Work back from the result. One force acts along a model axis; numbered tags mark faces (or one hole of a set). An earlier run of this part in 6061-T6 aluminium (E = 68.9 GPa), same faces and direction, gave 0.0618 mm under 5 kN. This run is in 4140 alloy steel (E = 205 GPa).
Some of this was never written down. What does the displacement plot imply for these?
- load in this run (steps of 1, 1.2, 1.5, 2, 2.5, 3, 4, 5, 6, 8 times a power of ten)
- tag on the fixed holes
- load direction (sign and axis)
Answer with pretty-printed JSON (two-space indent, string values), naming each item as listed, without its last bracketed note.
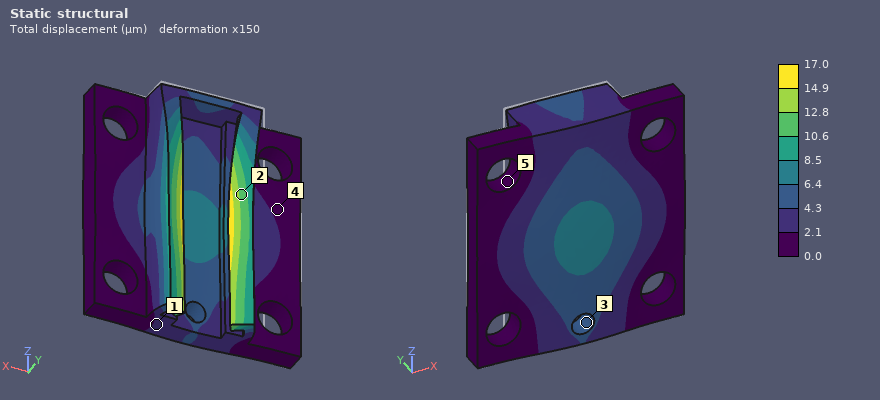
{
  "load in this run": "4 kN",
  "tag on the fixed holes": "5",
  "load direction": "-Y"
}
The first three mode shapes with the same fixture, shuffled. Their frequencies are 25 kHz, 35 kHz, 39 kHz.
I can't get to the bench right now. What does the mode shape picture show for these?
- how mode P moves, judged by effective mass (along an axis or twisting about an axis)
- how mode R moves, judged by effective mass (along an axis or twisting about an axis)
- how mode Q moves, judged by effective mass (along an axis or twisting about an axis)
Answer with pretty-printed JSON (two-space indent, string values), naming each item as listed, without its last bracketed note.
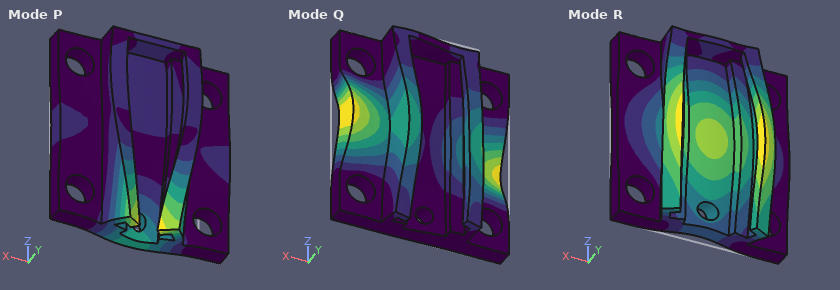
{
  "how mode P moves, judged by effective mass": "twisting about X",
  "how mode R moves, judged by effective mass": "along Y",
  "how mode Q moves, judged by effective mass": "twisting about Z"
}
